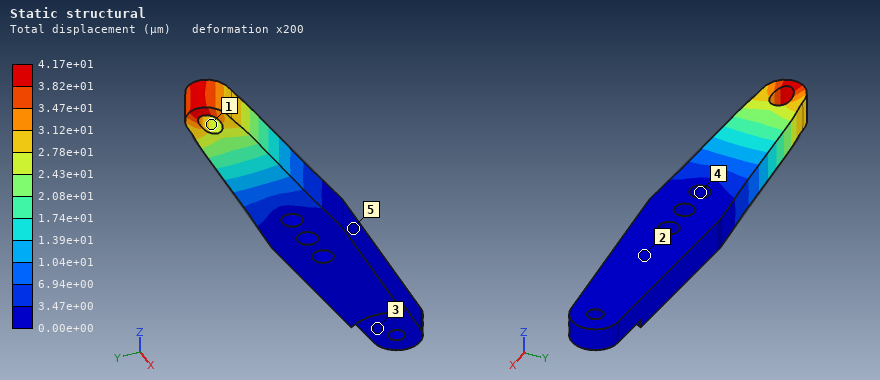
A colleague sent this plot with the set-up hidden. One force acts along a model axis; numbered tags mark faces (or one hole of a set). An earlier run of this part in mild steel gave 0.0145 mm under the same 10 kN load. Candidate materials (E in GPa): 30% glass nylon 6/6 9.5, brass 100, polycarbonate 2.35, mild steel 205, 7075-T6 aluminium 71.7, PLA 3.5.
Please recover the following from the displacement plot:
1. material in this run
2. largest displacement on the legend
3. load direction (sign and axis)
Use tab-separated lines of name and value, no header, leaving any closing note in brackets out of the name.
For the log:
material in this run	7075-T6 aluminium
largest displacement on the legend	4.17e+01 µm
load direction	-X
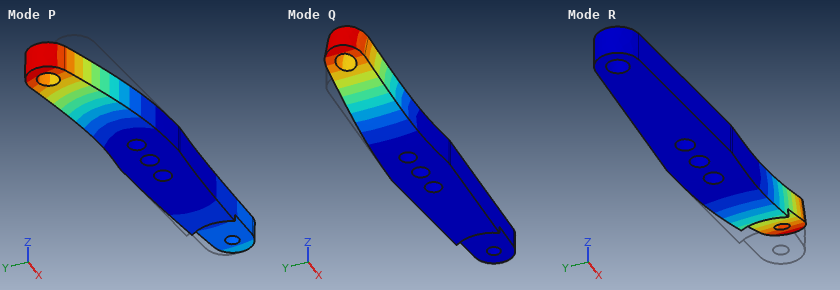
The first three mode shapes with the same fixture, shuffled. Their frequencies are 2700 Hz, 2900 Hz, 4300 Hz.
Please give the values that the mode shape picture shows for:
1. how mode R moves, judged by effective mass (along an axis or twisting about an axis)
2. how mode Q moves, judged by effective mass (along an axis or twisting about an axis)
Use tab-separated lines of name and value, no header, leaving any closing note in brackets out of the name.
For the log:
how mode R moves, judged by effective mass	along Z
how mode Q moves, judged by effective mass	along Z
